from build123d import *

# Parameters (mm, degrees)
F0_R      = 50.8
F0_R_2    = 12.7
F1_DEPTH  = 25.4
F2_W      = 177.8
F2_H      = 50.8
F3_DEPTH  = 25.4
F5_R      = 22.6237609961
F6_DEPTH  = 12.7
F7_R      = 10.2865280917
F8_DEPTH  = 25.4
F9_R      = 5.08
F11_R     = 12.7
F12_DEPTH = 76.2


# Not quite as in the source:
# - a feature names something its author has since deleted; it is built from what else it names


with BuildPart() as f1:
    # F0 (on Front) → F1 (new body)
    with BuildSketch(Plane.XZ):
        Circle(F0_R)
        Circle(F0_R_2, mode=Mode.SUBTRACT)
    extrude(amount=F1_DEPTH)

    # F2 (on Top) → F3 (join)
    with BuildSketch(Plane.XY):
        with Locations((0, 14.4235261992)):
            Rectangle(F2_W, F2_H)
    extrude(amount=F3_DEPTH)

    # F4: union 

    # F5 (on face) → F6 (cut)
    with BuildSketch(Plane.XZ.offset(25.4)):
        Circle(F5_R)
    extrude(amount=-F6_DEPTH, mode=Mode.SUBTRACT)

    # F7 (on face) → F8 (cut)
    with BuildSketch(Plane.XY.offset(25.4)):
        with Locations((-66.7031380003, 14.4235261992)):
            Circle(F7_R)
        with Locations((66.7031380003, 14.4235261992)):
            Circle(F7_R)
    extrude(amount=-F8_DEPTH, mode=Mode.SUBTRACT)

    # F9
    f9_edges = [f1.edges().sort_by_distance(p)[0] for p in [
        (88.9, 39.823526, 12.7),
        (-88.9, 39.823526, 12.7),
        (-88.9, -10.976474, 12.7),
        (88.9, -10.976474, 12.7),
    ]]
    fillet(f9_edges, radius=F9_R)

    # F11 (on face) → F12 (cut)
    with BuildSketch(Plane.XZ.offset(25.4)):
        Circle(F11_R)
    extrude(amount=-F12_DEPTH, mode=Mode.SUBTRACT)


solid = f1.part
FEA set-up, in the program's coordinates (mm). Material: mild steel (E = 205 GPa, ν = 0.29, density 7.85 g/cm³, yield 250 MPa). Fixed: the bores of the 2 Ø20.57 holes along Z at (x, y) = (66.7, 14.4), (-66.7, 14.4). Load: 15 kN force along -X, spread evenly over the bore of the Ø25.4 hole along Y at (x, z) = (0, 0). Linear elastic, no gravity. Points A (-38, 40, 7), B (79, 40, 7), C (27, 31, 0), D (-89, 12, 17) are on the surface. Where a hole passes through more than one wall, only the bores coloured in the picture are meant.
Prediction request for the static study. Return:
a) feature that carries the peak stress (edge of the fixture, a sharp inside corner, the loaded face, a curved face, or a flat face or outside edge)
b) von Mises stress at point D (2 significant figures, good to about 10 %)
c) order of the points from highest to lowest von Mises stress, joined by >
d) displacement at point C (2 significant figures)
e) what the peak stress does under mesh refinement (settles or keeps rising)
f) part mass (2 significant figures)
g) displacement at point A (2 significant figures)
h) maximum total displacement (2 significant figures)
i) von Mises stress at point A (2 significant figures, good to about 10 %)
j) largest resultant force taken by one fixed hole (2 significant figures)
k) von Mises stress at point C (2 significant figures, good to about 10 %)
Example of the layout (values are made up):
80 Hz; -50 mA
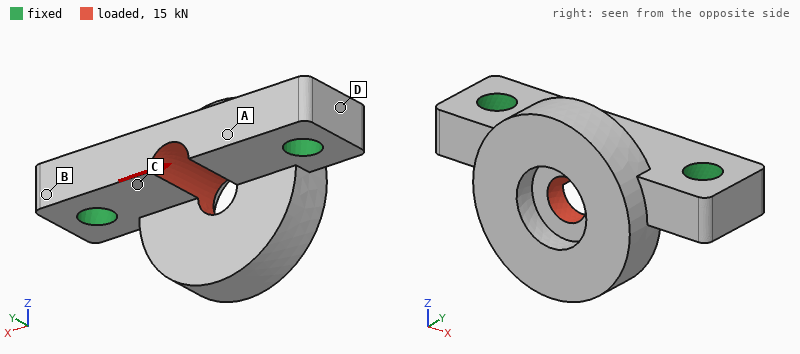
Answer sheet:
edge of the fixture; 2.5 MPa; C > A > D > B; 0.98 µm; keeps rising; 2.8 kg; 0.74 µm; 2.5 µm; 4.6 MPa; 7.6 kN; 6.3 MPa
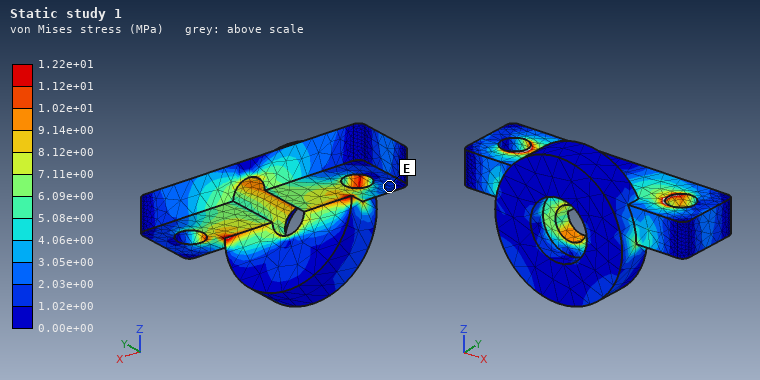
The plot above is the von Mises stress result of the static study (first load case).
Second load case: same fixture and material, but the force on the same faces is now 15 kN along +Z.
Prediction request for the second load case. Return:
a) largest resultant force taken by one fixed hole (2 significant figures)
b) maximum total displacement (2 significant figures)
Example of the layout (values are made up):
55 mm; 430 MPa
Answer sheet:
7.8 kN; 12 µm
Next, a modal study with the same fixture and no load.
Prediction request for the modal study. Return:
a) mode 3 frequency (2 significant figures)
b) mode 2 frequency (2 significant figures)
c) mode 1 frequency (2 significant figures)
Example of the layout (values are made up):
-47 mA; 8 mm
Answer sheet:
7000 Hz; 5900 Hz; 3000 Hz
